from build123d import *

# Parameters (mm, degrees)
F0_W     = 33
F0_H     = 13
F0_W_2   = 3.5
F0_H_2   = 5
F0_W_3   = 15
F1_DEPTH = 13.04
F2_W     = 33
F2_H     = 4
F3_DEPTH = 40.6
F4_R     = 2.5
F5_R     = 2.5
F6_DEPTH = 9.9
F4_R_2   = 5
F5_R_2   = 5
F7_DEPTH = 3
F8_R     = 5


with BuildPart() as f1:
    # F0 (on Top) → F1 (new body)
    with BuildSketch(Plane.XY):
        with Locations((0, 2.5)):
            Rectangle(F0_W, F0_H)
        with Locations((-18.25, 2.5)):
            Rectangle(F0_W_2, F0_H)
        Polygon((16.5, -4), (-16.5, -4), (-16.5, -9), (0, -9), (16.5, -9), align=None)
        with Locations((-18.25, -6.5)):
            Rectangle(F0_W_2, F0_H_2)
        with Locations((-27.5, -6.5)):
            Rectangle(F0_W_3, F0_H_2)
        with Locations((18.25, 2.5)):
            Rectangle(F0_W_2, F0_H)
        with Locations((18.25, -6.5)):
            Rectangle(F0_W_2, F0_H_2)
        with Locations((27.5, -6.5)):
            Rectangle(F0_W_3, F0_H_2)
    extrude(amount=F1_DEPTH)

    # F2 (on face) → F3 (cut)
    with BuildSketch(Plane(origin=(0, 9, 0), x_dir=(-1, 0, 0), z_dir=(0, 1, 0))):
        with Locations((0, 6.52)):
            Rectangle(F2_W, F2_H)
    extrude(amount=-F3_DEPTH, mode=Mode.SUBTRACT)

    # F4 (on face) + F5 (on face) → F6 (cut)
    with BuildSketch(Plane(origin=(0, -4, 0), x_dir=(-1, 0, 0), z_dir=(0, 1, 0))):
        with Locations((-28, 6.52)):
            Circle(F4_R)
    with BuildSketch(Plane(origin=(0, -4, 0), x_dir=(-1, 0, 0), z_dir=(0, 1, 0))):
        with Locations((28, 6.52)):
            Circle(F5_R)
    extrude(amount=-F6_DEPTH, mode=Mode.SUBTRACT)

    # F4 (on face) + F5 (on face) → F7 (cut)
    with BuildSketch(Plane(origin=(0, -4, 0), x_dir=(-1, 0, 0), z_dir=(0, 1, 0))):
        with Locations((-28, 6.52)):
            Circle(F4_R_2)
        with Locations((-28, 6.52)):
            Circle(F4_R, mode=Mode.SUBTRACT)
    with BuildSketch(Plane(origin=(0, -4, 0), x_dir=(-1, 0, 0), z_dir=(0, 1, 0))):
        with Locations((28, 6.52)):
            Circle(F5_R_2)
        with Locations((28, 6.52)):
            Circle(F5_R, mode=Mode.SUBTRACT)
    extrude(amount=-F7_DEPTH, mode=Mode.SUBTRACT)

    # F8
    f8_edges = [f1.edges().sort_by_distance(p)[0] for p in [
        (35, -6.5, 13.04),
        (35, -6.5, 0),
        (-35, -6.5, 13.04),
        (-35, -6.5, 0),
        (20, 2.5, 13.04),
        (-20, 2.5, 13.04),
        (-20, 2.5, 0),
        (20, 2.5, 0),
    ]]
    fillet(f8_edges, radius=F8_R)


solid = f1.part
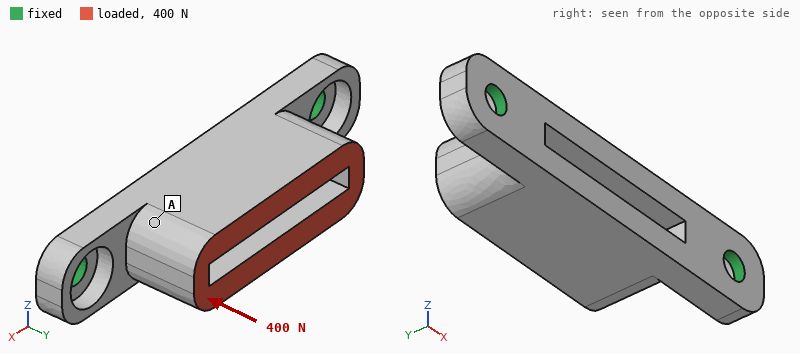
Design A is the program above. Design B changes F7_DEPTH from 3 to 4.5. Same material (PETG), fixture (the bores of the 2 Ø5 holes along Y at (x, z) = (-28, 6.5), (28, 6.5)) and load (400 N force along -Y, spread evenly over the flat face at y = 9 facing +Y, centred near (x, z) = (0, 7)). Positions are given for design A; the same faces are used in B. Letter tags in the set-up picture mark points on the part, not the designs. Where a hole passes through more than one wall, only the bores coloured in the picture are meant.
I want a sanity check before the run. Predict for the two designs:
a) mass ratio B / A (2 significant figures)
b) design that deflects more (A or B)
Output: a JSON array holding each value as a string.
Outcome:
["0.98", "B"]
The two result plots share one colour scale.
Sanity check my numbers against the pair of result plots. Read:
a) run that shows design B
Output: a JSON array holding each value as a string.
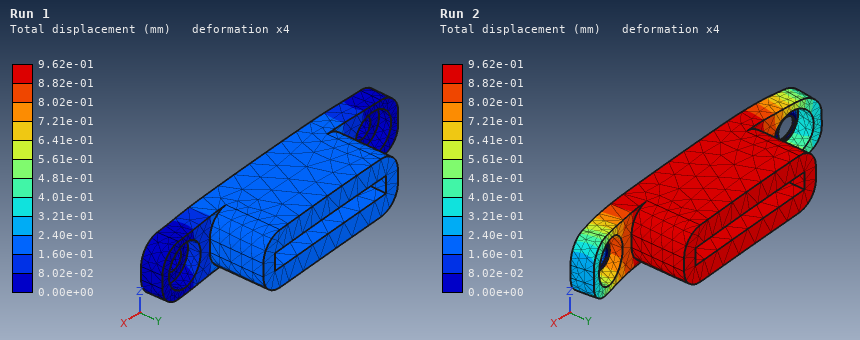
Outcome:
["Run 2"]
